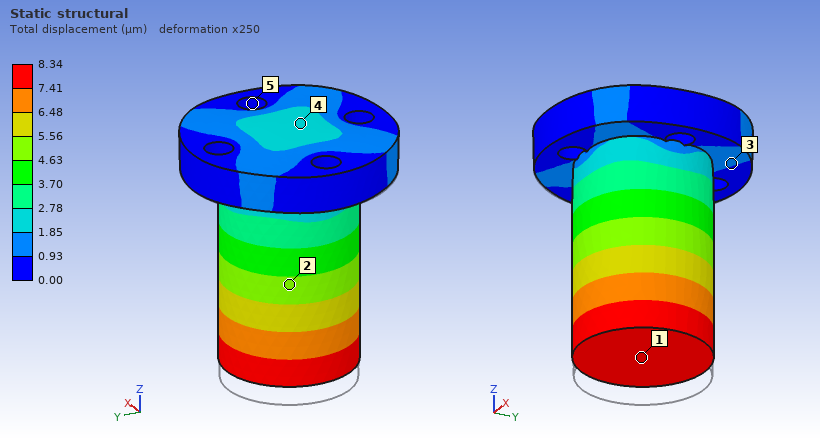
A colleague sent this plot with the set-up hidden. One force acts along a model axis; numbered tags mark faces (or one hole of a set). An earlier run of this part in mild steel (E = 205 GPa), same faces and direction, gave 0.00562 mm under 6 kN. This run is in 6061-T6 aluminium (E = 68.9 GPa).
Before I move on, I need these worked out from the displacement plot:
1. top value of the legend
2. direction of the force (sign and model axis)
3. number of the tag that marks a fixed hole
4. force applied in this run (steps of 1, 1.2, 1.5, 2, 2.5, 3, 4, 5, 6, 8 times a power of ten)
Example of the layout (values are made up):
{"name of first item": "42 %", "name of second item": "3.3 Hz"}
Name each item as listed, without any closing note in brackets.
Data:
{"top value of the legend": "8.34 µm", "direction of the force": "+Z", "number of the tag that marks a fixed hole": "5", "force applied in this run": "3 kN"}
